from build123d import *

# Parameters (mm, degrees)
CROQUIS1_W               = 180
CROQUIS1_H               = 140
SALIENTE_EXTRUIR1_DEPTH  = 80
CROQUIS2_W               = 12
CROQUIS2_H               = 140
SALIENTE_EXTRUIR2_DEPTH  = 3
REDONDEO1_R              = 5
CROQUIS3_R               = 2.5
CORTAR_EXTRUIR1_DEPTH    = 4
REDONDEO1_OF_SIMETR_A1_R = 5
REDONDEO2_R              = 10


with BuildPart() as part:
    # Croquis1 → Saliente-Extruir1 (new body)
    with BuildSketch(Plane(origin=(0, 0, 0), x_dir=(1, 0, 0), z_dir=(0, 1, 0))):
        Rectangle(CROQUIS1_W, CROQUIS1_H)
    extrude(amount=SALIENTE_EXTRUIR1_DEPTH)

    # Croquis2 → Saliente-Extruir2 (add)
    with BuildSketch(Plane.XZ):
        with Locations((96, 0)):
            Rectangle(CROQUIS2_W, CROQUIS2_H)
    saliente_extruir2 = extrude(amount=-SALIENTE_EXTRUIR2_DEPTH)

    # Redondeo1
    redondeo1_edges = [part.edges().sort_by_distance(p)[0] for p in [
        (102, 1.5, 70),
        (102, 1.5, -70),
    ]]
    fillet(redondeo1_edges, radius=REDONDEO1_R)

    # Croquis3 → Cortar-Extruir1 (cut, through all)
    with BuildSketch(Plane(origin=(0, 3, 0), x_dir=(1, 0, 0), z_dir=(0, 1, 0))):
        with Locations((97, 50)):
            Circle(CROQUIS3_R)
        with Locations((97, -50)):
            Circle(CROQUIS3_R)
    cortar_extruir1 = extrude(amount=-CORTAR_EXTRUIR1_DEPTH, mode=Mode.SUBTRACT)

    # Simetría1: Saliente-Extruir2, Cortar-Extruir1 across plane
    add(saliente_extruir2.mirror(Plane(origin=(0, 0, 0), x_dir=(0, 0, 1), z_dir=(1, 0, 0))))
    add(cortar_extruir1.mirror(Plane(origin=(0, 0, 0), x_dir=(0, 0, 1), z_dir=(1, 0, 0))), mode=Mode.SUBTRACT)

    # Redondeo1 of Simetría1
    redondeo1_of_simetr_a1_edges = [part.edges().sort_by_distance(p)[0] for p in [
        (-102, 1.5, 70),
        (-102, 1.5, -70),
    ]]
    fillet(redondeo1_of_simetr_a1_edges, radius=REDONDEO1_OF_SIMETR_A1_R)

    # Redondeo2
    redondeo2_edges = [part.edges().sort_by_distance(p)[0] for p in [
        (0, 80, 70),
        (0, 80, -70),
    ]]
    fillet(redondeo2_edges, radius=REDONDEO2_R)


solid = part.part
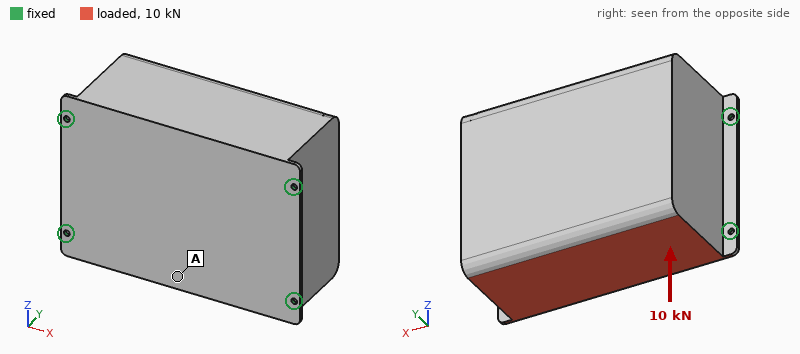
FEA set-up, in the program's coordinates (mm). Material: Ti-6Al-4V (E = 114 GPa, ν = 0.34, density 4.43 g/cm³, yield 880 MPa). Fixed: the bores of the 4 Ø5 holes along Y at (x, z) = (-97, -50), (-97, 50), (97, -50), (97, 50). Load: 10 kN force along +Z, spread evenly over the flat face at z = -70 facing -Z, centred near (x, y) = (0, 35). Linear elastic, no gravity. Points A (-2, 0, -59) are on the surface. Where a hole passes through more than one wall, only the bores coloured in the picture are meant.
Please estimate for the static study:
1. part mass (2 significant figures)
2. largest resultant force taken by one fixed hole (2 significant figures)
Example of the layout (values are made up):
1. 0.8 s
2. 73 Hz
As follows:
1. 8.9 kg
2. 3.2 kN
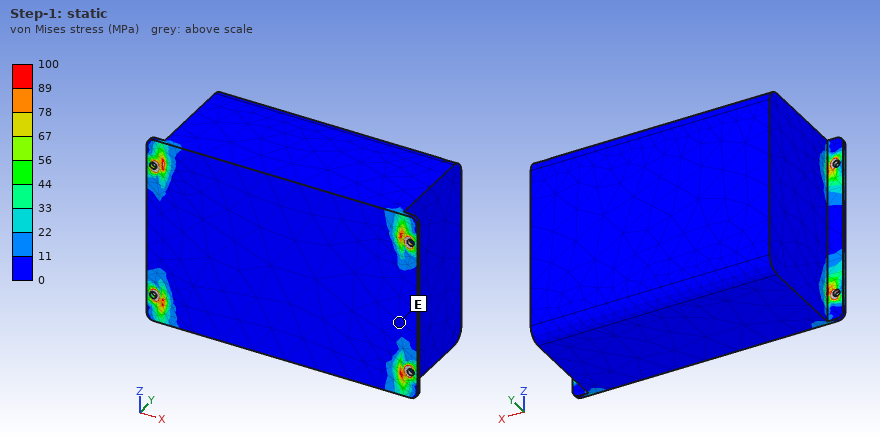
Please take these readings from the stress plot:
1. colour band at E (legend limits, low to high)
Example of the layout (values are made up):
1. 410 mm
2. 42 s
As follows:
1. 0 to 11 MPa
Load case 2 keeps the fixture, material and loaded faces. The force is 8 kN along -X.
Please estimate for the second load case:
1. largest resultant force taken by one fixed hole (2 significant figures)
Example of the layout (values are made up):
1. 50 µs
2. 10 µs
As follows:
1. 3.0 kN
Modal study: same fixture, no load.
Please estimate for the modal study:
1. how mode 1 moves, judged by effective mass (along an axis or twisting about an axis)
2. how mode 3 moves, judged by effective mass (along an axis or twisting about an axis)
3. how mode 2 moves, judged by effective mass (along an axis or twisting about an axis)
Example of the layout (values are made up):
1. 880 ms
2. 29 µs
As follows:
1. along Z
2. along X
3. along Y
